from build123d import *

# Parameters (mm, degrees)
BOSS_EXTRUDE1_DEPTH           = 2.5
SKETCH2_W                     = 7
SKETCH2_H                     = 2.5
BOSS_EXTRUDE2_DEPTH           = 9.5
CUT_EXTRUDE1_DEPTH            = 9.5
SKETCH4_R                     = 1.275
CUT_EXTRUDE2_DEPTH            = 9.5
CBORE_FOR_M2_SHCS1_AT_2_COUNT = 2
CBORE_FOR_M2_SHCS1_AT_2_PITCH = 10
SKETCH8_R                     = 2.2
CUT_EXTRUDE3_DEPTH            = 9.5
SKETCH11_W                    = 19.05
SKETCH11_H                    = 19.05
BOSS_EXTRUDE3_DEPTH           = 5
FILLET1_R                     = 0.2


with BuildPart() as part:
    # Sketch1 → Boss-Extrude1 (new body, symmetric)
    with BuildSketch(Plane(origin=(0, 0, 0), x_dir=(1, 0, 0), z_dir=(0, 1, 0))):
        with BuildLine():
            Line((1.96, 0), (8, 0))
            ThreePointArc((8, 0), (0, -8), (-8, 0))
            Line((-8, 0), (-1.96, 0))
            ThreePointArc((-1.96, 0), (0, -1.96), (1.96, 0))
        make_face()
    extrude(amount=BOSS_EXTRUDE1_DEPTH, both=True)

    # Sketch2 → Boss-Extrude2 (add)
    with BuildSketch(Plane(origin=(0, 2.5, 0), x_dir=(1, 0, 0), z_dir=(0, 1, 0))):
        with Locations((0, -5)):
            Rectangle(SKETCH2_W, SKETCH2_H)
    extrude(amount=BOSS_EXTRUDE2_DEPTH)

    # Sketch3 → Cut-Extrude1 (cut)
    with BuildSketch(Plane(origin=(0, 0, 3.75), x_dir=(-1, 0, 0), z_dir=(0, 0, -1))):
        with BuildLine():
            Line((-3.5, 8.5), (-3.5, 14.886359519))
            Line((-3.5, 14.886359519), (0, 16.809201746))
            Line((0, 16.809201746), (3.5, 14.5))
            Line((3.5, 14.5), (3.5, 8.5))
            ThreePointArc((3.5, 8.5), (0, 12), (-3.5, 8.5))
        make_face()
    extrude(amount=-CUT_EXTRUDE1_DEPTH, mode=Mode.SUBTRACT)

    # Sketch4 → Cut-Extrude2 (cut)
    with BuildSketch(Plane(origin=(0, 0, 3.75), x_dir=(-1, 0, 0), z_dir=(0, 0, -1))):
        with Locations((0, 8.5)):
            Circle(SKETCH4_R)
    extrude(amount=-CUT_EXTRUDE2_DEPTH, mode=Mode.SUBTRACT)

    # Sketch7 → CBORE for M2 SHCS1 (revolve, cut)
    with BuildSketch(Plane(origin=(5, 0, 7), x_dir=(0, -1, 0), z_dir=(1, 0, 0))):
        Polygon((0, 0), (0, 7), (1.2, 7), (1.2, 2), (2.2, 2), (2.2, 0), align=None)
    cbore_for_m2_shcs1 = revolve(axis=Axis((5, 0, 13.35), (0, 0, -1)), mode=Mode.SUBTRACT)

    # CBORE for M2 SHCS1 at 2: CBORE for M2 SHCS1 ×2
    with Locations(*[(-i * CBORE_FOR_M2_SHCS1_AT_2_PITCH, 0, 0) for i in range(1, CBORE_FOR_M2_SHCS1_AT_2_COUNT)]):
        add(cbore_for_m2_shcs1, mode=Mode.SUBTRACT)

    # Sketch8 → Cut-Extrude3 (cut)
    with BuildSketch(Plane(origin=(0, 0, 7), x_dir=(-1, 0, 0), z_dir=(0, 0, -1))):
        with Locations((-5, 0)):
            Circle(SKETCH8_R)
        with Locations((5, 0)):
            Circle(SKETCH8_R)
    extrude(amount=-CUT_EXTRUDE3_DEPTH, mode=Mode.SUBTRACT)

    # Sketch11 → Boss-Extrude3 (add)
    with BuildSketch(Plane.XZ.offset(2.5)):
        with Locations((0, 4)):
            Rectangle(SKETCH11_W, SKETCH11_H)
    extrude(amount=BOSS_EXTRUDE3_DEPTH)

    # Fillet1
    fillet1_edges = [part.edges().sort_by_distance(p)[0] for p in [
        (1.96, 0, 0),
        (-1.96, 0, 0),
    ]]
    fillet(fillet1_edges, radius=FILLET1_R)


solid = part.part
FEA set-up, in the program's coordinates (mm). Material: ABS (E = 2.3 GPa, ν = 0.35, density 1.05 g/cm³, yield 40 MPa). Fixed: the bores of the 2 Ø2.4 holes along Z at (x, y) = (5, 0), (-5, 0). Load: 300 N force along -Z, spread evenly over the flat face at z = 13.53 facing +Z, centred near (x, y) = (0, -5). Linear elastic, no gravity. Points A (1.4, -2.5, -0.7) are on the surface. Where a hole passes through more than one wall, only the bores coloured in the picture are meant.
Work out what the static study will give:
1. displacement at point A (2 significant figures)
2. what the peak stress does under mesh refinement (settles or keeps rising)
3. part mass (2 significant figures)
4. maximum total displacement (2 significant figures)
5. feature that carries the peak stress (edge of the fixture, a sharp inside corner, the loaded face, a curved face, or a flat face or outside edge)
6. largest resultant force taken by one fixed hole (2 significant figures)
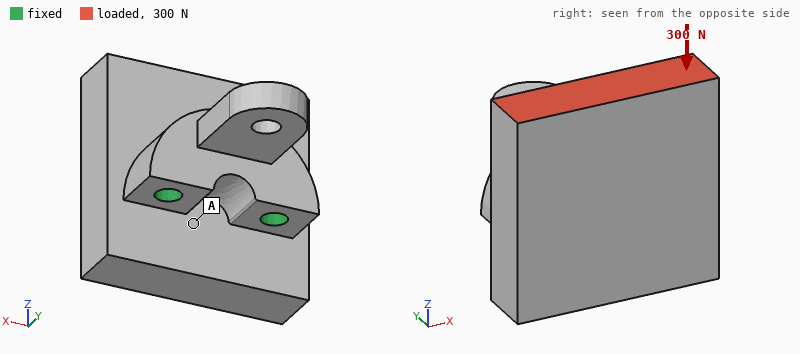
0.040 mm
keeps rising
2.5 g
0.15 mm
edge of the fixture
150 N
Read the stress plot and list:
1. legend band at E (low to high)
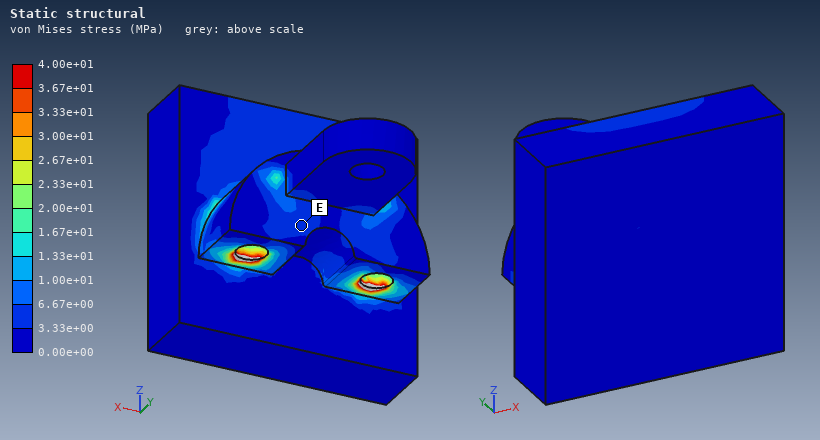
3.33e+00 to 6.67e+00 MPa
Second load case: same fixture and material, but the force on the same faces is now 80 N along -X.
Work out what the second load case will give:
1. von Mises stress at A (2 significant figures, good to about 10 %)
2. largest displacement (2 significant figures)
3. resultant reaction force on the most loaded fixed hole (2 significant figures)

1.4 MPa
51 µm
91 N
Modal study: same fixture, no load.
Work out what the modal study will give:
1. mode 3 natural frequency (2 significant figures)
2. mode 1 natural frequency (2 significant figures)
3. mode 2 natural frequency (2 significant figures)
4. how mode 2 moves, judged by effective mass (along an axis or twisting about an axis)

8500 Hz
5000 Hz
6600 Hz
along Z
